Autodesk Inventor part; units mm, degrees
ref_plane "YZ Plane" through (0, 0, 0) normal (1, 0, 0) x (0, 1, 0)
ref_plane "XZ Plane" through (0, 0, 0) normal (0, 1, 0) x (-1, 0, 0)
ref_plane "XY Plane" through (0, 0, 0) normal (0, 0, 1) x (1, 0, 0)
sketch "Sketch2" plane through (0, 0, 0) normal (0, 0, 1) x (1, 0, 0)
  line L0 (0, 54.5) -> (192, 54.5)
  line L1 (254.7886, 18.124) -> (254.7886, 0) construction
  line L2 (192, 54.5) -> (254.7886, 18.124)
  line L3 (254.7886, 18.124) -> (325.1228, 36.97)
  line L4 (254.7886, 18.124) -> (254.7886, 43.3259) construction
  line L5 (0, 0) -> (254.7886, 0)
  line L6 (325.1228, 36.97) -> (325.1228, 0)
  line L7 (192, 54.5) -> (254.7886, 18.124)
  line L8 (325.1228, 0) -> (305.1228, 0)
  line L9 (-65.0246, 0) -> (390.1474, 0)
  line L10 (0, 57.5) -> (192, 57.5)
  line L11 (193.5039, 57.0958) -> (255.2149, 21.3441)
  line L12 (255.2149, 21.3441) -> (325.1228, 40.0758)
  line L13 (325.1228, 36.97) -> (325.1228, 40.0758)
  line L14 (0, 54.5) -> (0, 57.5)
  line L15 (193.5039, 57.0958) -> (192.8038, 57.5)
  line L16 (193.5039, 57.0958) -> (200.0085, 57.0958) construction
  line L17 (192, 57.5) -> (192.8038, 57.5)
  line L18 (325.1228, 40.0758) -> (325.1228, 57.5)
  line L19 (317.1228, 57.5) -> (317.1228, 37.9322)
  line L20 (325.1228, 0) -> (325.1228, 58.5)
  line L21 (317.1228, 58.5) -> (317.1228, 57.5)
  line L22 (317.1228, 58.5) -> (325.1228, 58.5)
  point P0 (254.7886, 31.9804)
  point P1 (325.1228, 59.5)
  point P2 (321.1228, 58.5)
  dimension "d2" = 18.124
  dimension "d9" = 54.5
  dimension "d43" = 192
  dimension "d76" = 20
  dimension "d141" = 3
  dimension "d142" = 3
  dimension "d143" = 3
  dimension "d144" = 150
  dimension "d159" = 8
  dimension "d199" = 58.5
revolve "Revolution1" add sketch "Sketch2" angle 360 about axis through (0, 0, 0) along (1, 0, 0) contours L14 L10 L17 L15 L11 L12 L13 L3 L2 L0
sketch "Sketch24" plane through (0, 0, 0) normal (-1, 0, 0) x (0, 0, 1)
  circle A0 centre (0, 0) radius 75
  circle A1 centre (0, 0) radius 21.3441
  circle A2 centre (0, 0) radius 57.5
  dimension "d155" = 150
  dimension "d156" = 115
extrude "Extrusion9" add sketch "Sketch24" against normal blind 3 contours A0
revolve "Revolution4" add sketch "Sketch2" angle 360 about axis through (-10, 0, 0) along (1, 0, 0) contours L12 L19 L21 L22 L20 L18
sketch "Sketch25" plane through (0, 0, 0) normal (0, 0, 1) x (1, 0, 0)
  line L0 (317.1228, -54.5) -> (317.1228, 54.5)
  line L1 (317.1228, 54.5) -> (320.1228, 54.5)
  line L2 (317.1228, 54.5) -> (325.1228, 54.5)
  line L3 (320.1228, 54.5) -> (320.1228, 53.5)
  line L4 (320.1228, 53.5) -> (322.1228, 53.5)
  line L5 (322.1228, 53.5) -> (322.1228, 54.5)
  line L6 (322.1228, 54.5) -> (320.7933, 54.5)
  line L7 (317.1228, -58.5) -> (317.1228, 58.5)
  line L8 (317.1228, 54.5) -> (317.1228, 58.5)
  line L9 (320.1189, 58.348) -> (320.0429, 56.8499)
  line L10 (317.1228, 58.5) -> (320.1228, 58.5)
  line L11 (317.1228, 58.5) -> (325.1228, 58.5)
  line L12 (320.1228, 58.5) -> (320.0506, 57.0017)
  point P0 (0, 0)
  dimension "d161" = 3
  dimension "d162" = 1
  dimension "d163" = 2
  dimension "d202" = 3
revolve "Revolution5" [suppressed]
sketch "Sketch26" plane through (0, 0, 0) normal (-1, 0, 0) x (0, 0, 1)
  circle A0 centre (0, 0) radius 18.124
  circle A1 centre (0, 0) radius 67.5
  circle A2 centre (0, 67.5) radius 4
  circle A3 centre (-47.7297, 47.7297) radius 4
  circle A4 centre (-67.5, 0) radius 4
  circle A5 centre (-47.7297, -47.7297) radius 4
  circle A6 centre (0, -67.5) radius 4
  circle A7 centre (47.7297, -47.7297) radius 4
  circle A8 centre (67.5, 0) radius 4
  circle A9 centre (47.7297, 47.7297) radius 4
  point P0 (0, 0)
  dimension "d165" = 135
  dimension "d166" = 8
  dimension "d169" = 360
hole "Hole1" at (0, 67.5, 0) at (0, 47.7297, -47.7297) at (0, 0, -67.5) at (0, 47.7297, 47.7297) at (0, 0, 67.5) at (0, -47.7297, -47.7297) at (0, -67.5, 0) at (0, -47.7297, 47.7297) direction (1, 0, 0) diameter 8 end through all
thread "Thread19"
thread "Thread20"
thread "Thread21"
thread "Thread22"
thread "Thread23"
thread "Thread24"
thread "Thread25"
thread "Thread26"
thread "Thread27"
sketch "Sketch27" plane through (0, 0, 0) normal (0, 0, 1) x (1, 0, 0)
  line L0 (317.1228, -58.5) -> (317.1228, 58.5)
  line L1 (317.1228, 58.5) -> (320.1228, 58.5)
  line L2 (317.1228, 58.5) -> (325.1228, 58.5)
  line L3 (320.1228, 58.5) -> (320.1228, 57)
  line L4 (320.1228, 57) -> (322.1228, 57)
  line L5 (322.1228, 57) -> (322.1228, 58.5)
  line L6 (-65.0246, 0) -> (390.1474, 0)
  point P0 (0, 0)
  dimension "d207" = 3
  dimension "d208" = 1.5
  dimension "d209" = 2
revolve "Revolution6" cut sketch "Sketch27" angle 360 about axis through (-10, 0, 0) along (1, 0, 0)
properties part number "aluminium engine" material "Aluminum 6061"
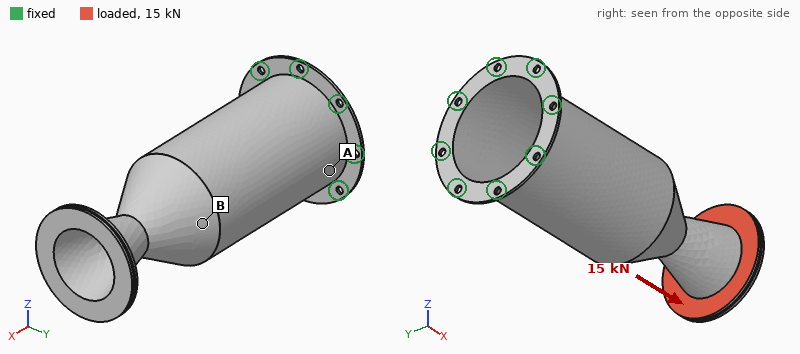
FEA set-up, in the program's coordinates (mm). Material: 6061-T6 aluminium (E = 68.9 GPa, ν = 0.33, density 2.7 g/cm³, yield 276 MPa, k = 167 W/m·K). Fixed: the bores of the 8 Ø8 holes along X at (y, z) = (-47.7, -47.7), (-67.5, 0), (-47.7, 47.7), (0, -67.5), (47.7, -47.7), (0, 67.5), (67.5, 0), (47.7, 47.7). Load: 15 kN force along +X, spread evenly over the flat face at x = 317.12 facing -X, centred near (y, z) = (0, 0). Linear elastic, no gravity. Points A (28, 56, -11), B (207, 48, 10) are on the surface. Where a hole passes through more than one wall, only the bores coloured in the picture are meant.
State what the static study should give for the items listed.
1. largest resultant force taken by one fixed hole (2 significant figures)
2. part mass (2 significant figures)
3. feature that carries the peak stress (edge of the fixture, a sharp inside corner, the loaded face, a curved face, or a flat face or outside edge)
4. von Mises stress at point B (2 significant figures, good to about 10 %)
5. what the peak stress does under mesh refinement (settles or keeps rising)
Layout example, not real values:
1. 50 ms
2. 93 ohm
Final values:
1. 2.0 kN
2. 980 g
3. edge of the fixture
4. 29 MPa
5. keeps rising
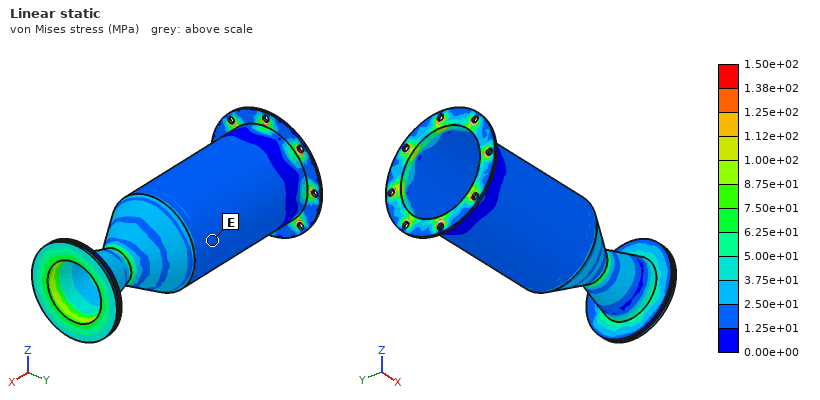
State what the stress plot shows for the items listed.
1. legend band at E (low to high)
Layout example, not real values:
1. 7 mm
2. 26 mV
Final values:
1. 1.25e+01 to 2.50e+01 MPa
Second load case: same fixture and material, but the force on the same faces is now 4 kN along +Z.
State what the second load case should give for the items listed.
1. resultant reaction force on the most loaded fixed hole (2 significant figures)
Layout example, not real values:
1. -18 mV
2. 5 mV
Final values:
1. 5.5 kN
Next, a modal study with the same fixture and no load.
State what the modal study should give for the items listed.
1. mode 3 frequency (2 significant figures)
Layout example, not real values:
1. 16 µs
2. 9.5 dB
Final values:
1. 1800 Hz
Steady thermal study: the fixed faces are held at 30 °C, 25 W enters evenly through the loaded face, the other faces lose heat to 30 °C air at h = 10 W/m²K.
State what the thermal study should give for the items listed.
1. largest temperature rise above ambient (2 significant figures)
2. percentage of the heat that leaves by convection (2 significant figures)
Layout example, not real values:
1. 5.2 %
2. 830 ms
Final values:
1. 32 K
2. 77 %
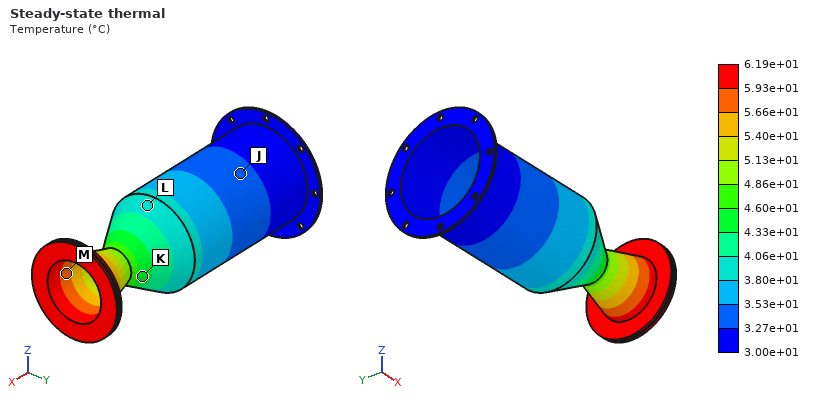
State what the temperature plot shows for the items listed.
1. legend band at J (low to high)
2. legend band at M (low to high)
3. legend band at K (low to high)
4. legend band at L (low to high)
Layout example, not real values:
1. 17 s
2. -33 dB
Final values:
1. 3.27e+01 to 3.53e+01 °C
2. 5.66e+01 to 5.93e+01 °C
3. 4.33e+01 to 4.60e+01 °C
4. 3.80e+01 to 4.06e+01 °C
